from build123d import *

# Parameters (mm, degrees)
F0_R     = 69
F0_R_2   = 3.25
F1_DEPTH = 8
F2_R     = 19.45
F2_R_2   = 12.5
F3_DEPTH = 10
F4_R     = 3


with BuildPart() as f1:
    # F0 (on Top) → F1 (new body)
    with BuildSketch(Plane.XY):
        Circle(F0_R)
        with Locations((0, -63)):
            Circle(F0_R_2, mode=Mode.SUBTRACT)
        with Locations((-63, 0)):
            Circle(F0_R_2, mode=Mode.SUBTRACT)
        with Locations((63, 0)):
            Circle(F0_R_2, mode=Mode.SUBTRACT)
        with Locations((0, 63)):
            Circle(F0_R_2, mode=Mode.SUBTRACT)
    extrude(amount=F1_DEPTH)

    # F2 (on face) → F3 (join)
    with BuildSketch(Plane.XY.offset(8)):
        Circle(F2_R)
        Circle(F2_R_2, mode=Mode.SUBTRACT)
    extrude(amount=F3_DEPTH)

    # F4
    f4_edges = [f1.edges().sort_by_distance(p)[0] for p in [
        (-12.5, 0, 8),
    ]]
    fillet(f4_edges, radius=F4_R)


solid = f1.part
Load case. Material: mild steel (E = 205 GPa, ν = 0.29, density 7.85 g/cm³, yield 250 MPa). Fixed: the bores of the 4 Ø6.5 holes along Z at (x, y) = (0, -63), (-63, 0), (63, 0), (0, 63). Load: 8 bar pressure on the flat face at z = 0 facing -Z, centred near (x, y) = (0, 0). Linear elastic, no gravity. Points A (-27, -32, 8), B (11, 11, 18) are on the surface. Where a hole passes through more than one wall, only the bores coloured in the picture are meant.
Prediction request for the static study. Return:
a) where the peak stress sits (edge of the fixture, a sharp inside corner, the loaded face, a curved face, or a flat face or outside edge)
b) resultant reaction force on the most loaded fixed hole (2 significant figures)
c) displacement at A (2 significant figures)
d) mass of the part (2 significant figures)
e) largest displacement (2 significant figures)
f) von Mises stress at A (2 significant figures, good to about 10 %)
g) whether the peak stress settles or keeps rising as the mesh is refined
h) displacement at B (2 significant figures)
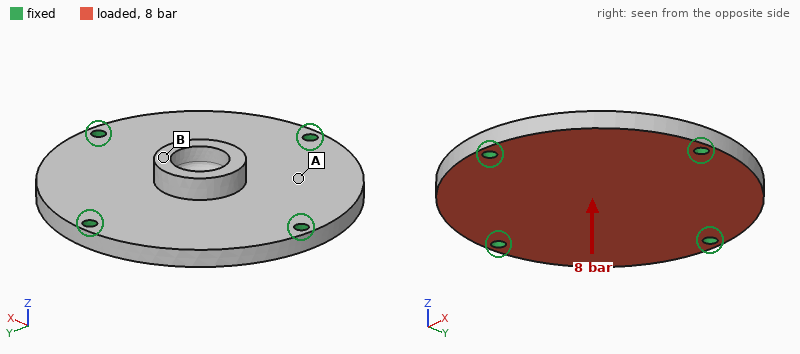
edge of the fixture
3.0 kN
25 µm
990 g
33 µm
29 MPa
keeps rising
32 µm
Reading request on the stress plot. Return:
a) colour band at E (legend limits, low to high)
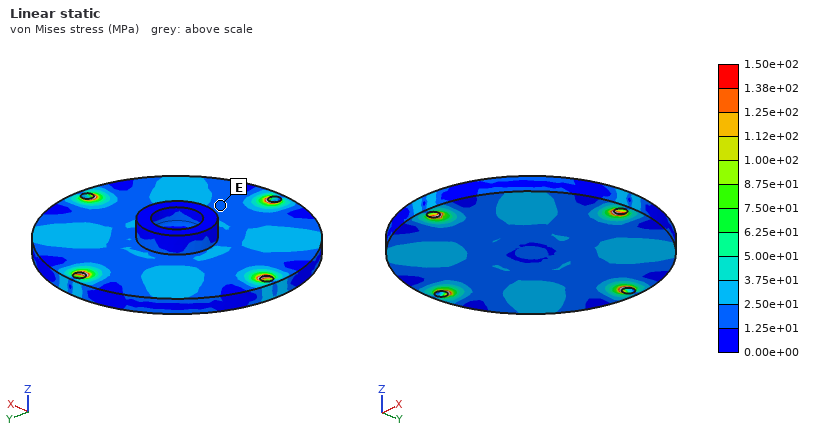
1.25e+01 to 2.50e+01 MPa
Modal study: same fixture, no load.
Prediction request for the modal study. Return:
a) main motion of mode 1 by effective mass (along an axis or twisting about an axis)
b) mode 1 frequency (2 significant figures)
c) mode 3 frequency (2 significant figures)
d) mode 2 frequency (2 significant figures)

along Z
3400 Hz
4500 Hz
4400 Hz
